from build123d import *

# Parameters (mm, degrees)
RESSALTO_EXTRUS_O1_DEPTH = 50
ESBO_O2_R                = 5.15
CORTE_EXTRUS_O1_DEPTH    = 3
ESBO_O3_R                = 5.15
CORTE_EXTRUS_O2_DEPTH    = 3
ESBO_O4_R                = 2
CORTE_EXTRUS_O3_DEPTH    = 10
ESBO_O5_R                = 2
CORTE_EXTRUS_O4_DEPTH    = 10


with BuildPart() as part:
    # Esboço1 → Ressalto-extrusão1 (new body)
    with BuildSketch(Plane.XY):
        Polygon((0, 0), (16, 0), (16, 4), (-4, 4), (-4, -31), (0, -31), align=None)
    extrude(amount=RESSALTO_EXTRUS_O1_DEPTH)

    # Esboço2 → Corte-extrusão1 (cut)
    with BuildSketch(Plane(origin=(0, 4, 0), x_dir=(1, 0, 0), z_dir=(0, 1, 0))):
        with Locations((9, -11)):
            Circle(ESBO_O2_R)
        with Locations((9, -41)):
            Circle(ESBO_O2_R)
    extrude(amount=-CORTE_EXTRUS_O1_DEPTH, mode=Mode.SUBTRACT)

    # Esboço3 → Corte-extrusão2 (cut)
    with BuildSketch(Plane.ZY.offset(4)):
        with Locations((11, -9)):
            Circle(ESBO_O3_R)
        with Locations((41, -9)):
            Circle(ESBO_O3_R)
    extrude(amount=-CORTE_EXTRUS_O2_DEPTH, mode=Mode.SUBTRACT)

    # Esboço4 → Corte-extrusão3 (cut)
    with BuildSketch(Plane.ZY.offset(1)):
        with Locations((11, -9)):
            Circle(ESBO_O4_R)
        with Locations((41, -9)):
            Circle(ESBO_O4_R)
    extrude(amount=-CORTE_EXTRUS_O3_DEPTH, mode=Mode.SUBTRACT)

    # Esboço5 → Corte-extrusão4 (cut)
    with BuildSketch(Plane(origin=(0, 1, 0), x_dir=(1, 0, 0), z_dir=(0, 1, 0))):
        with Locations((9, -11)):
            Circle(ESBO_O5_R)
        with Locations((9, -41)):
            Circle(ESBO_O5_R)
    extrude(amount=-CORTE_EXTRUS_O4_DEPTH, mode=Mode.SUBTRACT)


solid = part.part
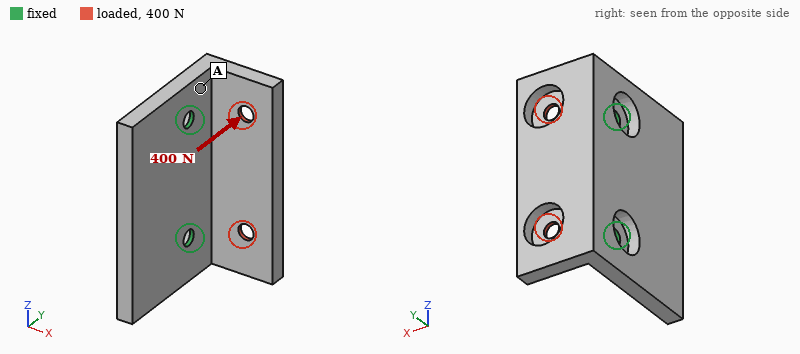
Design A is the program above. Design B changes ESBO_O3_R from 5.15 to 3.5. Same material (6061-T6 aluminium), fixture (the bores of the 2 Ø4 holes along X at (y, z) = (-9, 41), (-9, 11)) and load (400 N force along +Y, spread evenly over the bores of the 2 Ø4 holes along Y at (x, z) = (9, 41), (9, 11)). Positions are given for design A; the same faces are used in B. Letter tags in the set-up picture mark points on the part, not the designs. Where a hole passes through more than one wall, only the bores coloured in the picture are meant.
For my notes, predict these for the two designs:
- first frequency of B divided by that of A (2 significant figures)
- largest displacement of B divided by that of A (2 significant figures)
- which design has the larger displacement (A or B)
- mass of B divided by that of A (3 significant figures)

1.3
0.68
A
1.03
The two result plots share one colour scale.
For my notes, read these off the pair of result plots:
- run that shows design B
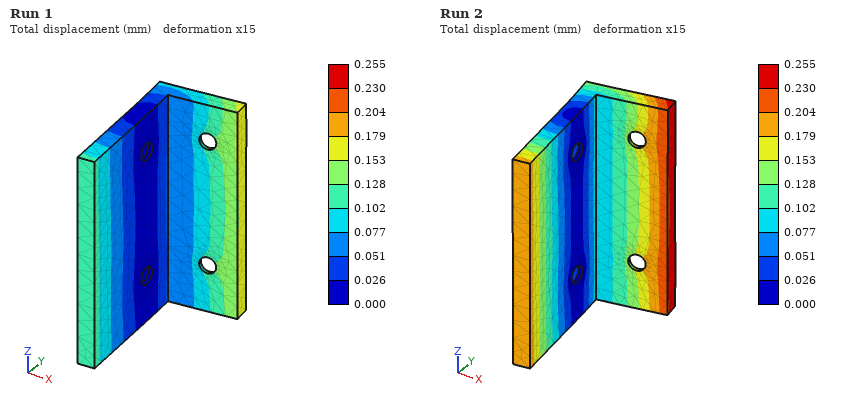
Run 1
